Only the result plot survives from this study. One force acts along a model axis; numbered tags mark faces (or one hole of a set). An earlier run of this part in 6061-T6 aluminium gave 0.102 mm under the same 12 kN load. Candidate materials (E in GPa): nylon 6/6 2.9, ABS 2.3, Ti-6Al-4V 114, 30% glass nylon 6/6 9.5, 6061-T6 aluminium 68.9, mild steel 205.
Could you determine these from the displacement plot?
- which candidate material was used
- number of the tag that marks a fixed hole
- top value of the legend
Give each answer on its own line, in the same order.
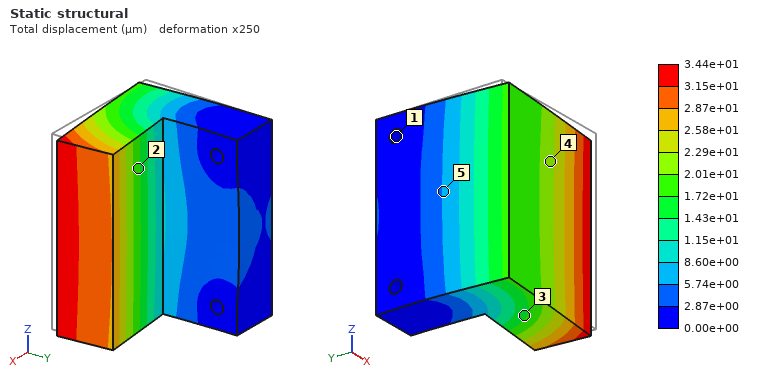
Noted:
mild steel
1
3.44e+01 µm
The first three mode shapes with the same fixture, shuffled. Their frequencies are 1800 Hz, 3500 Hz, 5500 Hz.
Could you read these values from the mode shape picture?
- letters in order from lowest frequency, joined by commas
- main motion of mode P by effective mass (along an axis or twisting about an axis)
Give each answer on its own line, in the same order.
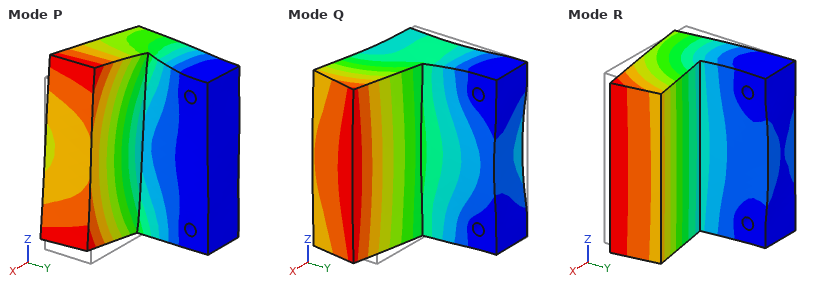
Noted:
R, P, Q
along Z
